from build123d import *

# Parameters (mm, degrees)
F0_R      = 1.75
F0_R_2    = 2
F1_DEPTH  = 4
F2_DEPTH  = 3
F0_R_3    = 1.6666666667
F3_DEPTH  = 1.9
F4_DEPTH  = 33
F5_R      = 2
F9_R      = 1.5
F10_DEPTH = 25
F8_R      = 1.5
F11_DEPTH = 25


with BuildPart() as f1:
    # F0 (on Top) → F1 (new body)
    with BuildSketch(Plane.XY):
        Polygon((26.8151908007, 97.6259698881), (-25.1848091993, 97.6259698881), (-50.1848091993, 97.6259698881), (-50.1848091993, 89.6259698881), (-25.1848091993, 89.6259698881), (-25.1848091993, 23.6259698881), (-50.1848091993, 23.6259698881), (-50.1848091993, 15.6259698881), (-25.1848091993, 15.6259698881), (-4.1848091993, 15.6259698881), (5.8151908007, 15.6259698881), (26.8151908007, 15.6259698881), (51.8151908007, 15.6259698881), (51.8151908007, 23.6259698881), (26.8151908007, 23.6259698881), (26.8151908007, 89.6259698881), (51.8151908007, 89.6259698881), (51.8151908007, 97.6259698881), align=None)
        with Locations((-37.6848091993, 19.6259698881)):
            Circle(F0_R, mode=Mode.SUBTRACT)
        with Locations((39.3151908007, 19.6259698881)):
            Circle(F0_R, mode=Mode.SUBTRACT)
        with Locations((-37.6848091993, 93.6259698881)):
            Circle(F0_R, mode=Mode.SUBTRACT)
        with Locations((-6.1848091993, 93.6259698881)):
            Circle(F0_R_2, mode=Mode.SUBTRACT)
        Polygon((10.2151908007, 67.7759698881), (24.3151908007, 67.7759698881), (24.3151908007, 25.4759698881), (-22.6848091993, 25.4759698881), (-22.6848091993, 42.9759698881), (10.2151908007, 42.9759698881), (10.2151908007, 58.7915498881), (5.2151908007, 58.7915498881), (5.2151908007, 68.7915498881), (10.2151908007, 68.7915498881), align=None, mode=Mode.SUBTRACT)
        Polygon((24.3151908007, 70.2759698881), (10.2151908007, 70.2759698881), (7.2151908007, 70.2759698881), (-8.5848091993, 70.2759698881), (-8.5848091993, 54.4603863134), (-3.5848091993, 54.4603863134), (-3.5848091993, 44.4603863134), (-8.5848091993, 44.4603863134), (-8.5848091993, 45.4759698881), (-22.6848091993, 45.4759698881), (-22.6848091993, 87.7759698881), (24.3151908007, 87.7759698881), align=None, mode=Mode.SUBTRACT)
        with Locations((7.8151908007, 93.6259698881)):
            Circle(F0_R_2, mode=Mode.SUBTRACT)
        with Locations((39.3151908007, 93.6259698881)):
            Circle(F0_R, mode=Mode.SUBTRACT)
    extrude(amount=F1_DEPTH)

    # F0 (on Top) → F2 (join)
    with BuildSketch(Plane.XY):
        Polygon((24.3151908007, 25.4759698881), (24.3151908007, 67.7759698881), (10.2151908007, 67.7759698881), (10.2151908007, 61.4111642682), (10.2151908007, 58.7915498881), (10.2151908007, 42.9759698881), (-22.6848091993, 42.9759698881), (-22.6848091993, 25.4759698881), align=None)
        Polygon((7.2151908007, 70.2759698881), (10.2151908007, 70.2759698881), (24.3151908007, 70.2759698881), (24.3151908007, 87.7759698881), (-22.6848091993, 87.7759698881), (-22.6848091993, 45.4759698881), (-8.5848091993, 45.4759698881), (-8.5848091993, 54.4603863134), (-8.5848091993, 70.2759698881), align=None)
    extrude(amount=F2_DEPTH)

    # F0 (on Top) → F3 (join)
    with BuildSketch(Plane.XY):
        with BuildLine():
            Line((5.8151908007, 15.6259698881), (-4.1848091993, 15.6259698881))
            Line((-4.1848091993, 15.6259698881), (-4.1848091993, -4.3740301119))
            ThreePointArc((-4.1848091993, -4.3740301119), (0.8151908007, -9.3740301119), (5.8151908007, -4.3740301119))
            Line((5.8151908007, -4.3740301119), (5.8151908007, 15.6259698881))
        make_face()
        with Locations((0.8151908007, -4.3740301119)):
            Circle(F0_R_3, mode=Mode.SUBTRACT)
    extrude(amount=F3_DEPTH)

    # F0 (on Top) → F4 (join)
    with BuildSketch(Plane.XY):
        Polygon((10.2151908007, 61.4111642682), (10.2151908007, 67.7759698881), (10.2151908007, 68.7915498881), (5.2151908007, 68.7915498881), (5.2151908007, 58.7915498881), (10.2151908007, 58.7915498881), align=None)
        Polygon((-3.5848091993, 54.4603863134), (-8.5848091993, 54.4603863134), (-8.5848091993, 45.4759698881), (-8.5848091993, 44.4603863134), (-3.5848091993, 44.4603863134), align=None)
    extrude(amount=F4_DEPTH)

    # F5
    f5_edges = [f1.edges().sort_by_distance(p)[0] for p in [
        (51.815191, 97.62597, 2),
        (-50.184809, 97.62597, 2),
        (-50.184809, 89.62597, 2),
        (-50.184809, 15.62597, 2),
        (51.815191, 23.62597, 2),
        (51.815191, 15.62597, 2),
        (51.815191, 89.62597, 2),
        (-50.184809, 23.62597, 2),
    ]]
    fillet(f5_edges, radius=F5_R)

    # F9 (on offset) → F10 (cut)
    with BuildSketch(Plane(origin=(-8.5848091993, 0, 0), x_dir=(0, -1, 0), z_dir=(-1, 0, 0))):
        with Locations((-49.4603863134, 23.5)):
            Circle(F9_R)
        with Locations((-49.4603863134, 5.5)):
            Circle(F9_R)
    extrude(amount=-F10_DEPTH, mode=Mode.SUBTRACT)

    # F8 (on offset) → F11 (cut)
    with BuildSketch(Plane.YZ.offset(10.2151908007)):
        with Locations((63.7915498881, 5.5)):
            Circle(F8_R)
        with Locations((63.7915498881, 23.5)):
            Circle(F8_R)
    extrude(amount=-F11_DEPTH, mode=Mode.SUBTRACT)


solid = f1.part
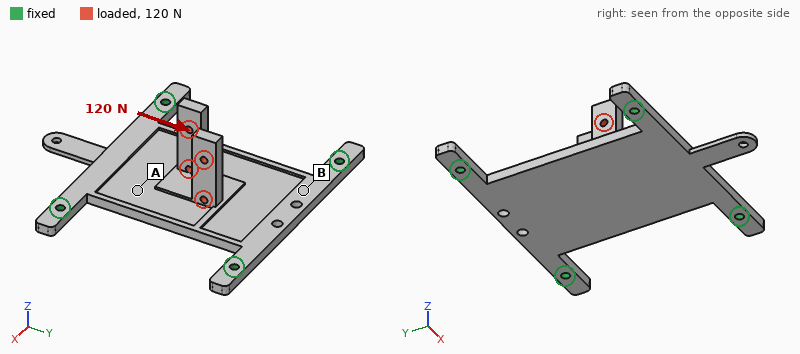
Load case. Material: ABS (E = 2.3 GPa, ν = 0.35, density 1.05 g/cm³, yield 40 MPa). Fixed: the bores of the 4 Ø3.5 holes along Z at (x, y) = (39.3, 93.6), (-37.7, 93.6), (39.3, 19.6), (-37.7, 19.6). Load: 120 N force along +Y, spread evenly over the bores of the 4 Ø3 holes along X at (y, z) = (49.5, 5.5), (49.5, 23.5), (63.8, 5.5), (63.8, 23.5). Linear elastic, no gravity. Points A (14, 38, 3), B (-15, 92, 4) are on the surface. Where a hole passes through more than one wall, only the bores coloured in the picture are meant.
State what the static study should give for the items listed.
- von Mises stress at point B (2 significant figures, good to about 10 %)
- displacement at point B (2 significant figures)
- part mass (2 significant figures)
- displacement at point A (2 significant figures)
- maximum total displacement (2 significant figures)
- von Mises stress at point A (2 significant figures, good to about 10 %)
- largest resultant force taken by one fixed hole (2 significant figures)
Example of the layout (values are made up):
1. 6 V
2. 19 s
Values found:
1. 1.6 MPa
2. 0.20 mm
3. 22 g
4. 0.24 mm
5. 0.93 mm
6. 3.5 MPa
7. 36 N
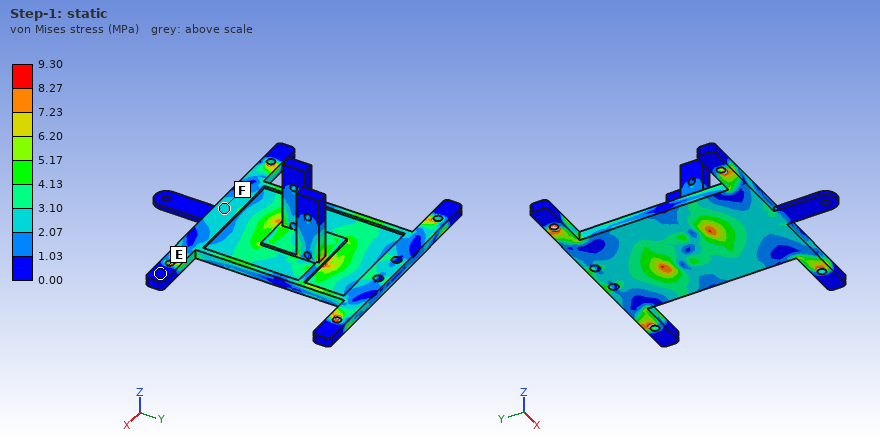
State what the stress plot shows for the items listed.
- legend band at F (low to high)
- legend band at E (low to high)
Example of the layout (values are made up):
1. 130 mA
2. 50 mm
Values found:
1. 2.07 to 3.10 MPa
2. 0.00 to 1.03 MPa
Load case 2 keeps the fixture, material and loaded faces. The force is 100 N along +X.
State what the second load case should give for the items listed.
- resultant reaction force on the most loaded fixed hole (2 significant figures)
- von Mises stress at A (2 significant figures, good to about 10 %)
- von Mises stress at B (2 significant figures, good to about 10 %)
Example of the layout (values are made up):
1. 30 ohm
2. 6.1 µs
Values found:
1. 28 N
2. 3.7 MPa
3. 3.1 MPa
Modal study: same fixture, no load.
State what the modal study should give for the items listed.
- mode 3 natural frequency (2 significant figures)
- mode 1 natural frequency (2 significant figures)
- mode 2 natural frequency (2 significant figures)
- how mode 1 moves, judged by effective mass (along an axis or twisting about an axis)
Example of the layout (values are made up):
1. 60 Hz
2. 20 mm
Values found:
1. 670 Hz
2. 420 Hz
3. 620 Hz
4. along Z
